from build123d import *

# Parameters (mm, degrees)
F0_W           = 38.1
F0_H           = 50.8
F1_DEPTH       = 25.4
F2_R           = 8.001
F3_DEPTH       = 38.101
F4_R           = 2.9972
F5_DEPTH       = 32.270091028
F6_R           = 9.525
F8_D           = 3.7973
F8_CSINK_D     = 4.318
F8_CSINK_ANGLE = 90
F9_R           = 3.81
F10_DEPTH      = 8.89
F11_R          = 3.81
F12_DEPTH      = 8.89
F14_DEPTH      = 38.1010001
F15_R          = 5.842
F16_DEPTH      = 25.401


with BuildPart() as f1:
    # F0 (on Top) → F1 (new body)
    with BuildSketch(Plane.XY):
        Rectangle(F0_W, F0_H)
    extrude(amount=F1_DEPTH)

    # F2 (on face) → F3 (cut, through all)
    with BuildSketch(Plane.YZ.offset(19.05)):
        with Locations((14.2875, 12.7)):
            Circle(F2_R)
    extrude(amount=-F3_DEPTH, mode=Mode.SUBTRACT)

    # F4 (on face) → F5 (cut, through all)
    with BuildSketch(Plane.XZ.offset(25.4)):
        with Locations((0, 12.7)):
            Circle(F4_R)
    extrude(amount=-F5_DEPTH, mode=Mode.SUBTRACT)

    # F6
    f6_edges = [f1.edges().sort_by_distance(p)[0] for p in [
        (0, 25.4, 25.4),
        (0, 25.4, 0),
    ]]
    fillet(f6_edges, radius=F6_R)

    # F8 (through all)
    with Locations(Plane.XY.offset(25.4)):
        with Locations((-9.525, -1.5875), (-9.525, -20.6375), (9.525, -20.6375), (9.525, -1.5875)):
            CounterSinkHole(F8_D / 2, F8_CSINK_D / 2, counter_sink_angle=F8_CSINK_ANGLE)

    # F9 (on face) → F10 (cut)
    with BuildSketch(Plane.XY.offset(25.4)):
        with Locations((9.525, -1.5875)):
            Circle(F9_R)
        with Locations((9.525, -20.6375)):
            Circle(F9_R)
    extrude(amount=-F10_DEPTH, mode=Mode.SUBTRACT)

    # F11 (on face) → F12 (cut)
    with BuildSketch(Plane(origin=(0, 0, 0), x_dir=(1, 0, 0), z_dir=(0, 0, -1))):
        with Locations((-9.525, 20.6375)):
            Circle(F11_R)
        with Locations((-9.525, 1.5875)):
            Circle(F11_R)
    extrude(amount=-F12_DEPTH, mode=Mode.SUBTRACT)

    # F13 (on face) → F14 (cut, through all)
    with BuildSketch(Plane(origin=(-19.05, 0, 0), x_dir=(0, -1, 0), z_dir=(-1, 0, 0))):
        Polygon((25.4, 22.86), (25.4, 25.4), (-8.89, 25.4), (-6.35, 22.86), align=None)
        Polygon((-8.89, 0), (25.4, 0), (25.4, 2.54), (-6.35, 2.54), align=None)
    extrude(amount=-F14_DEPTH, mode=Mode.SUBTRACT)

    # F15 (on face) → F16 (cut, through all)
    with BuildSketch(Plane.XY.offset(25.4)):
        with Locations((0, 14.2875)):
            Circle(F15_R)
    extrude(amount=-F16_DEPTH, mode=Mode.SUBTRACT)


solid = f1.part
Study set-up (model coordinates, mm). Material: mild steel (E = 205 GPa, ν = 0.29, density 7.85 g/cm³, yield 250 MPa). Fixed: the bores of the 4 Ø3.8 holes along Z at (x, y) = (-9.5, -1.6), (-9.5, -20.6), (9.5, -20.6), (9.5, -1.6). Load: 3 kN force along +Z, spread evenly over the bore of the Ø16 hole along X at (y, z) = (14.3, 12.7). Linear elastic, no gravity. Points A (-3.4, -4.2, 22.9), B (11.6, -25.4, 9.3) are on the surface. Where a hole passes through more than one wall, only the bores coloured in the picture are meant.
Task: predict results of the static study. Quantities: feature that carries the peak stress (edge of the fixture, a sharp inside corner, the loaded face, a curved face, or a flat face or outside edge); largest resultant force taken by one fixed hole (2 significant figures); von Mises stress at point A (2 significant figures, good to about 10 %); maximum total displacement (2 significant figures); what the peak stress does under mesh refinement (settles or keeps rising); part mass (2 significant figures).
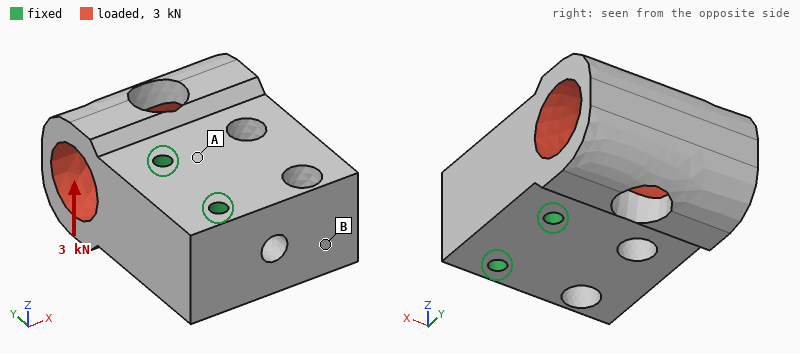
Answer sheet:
edge of the fixture
2.0 kN
13 MPa
13 µm
keeps rising
230 g
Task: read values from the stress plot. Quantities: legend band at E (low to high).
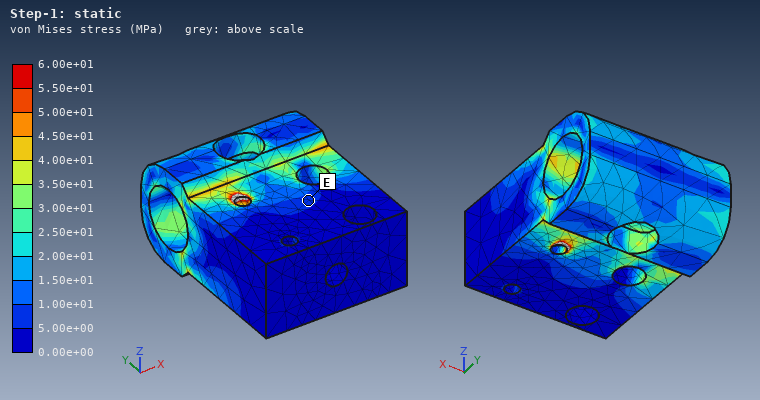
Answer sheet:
5.00e+00 to 1.00e+01 MPa
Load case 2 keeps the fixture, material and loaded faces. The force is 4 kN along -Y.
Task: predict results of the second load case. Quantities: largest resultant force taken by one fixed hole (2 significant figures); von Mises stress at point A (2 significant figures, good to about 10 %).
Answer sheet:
1.5 kN
4.4 MPa
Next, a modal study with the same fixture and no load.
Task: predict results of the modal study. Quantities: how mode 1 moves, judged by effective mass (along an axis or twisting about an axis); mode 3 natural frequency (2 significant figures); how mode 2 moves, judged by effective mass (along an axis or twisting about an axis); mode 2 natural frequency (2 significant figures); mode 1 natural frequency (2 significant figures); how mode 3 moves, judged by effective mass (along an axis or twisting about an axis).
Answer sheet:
along Z
18 kHz
along X
15 kHz
9800 Hz
twisting about Y
